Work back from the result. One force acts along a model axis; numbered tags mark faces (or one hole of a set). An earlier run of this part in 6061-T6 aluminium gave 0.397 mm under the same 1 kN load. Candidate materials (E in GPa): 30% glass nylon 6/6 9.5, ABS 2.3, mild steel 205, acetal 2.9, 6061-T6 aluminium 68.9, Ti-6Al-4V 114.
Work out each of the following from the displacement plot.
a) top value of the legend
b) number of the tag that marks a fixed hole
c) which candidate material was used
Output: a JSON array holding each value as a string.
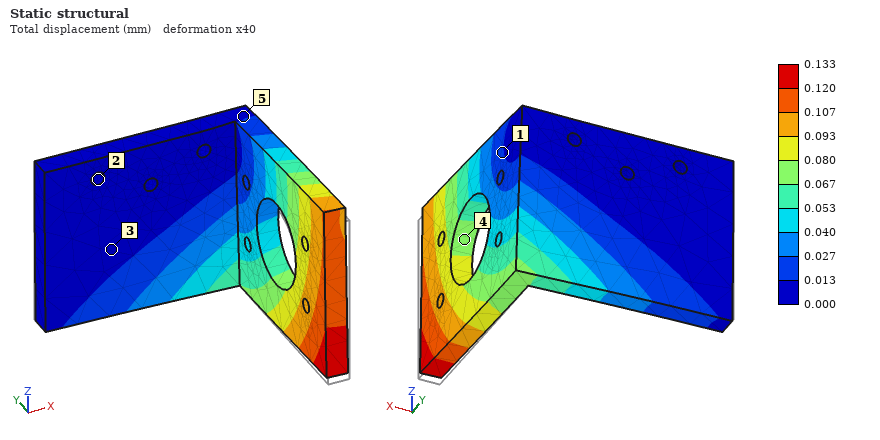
["0.133 mm", "2", "mild steel"]
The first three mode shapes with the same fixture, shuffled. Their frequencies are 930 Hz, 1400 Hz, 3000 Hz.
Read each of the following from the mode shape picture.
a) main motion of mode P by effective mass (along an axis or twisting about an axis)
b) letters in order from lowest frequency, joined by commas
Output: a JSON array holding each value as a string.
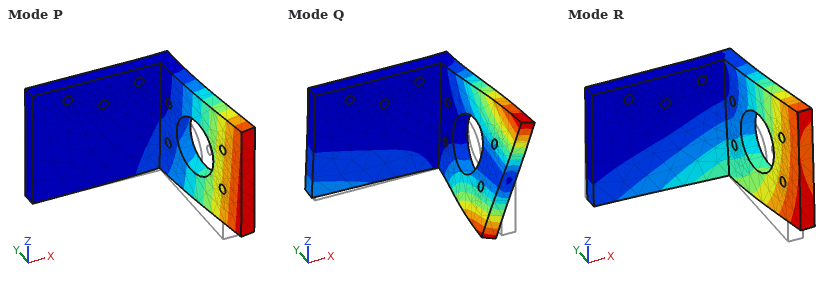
["along X", "P, R, Q"]
